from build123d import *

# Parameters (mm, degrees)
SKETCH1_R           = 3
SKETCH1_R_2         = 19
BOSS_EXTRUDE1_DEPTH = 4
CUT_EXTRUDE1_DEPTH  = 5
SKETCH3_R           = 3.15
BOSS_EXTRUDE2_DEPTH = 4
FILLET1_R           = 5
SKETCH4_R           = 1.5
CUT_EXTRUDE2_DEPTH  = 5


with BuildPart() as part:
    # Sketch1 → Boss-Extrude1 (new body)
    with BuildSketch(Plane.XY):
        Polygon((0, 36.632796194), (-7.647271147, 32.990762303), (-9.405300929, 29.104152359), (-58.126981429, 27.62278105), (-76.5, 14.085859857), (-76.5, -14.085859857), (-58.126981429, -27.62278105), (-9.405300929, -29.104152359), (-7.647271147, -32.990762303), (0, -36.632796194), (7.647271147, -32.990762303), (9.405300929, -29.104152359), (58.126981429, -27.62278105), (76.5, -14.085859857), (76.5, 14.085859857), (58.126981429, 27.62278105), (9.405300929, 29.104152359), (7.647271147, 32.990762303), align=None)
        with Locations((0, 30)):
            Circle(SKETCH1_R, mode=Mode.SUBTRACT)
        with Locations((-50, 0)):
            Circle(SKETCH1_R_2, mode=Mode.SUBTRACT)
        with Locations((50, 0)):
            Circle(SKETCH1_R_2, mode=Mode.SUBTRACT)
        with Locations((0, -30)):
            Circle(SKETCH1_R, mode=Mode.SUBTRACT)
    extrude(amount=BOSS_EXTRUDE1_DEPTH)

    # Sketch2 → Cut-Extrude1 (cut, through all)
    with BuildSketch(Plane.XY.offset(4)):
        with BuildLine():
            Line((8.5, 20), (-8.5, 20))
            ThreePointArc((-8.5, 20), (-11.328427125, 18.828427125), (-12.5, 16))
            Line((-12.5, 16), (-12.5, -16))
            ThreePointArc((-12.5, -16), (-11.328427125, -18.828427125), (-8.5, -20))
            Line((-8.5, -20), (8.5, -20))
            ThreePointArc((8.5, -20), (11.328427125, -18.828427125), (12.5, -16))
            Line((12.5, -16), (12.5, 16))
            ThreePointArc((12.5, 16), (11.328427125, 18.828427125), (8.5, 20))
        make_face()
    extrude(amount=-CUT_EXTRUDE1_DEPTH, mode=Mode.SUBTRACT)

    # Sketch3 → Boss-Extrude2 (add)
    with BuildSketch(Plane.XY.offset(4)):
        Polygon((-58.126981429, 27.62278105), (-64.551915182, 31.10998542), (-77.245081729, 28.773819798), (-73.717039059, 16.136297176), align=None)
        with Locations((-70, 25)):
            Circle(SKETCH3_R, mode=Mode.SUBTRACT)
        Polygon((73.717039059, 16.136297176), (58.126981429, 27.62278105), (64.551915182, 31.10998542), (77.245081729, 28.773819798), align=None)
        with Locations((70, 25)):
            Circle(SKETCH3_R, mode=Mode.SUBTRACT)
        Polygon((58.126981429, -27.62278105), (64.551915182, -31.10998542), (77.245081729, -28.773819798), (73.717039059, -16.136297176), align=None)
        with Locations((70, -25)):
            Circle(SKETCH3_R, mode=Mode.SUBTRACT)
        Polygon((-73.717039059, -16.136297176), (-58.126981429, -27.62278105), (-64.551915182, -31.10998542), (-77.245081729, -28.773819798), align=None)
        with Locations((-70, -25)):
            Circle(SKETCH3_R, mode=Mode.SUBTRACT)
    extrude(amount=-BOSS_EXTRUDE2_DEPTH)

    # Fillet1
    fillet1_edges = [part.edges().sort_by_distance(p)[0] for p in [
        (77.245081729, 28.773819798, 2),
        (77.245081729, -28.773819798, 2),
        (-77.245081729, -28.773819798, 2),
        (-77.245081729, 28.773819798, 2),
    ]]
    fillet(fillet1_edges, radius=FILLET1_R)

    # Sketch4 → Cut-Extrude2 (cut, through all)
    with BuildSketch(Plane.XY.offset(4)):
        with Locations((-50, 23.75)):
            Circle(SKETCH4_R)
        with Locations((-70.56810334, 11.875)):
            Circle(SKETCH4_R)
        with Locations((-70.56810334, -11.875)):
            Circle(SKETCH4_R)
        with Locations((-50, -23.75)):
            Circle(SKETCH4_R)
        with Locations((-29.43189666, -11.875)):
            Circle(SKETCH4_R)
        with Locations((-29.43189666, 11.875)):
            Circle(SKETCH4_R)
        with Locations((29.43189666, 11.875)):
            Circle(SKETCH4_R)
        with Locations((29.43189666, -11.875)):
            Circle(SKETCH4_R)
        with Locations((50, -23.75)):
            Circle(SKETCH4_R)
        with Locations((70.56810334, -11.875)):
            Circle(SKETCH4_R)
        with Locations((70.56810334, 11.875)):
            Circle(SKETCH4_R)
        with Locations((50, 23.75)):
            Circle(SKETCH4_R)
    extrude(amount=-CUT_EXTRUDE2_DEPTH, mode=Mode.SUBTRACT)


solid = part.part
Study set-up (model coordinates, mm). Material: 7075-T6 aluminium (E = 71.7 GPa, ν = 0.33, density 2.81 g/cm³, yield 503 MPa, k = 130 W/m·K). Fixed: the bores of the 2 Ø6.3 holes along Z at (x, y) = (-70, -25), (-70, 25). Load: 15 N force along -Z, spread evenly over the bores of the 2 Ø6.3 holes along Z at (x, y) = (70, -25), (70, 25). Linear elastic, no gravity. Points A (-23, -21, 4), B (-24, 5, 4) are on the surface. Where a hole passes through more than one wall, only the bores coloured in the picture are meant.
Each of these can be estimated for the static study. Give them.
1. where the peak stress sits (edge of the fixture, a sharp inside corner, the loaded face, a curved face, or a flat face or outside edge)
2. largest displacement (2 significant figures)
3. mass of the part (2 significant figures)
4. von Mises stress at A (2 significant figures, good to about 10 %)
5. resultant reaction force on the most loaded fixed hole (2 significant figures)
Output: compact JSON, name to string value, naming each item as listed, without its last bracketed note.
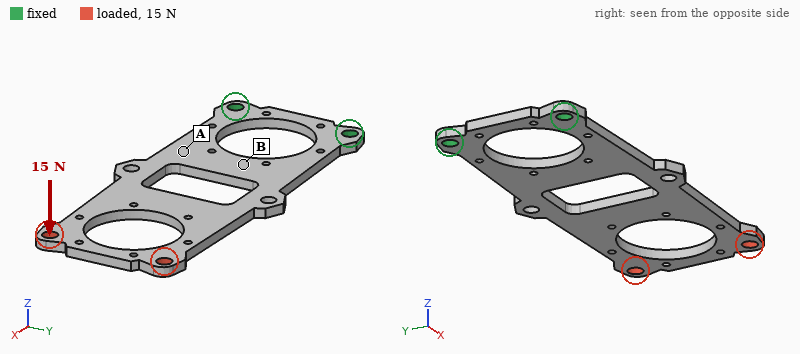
{"where the peak stress sits": "a curved face", "largest displacement": "1.6 mm", "mass of the part": "61 g", "von Mises stress at A": "14 MPa", "resultant reaction force on the most loaded fixed hole": "7.5 N"}
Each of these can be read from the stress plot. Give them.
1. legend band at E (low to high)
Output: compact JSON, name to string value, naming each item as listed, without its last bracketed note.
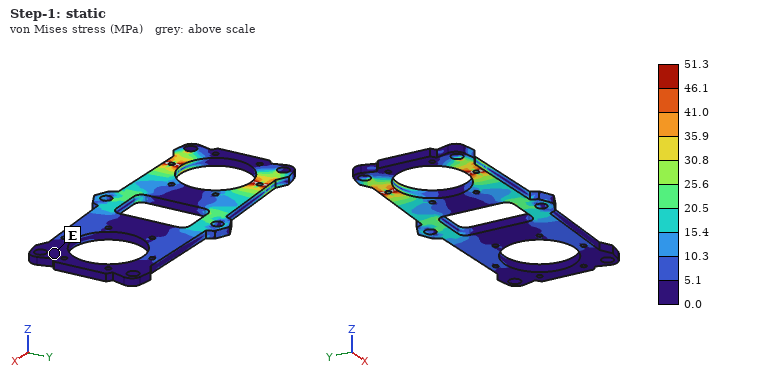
{"legend band at E": "0.0 to 5.1 MPa"}
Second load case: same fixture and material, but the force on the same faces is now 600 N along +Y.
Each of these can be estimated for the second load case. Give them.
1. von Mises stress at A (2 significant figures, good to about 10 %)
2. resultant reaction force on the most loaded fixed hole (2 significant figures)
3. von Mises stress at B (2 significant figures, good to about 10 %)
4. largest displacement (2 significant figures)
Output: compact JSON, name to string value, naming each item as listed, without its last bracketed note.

{"von Mises stress at A": "18 MPa", "resultant reaction force on the most loaded fixed hole": "1.6 kN", "von Mises stress at B": "20 MPa", "largest displacement": "0.35 mm"}
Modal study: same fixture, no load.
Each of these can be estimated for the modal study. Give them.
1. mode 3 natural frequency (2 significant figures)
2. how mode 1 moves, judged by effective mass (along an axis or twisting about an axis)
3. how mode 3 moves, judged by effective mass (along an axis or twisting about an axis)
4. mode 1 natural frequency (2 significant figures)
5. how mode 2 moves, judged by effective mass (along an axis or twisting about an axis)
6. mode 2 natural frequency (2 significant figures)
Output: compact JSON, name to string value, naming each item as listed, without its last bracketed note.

{"mode 3 natural frequency": "760 Hz", "how mode 1 moves, judged by effective mass": "along Z", "how mode 3 moves, judged by effective mass": "along Z", "mode 1 natural frequency": "130 Hz", "how mode 2 moves, judged by effective mass": "twisting about X", "mode 2 natural frequency": "650 Hz"}
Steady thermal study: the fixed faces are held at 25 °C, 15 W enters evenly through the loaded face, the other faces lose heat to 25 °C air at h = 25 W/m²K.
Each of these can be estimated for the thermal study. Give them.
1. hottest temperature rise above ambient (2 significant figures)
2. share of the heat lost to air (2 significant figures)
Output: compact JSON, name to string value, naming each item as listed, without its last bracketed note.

{"hottest temperature rise above ambient": "83 K", "share of the heat lost to air": "74 %"}
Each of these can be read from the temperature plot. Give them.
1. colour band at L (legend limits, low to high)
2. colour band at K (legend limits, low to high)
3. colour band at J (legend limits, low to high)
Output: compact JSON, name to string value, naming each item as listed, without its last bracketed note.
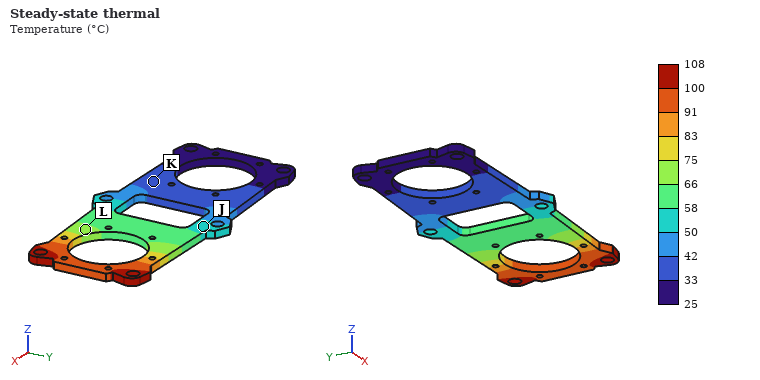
{"colour band at L": "66 to 75 °C", "colour band at K": "33 to 42 °C", "colour band at J": "50 to 58 °C"}
